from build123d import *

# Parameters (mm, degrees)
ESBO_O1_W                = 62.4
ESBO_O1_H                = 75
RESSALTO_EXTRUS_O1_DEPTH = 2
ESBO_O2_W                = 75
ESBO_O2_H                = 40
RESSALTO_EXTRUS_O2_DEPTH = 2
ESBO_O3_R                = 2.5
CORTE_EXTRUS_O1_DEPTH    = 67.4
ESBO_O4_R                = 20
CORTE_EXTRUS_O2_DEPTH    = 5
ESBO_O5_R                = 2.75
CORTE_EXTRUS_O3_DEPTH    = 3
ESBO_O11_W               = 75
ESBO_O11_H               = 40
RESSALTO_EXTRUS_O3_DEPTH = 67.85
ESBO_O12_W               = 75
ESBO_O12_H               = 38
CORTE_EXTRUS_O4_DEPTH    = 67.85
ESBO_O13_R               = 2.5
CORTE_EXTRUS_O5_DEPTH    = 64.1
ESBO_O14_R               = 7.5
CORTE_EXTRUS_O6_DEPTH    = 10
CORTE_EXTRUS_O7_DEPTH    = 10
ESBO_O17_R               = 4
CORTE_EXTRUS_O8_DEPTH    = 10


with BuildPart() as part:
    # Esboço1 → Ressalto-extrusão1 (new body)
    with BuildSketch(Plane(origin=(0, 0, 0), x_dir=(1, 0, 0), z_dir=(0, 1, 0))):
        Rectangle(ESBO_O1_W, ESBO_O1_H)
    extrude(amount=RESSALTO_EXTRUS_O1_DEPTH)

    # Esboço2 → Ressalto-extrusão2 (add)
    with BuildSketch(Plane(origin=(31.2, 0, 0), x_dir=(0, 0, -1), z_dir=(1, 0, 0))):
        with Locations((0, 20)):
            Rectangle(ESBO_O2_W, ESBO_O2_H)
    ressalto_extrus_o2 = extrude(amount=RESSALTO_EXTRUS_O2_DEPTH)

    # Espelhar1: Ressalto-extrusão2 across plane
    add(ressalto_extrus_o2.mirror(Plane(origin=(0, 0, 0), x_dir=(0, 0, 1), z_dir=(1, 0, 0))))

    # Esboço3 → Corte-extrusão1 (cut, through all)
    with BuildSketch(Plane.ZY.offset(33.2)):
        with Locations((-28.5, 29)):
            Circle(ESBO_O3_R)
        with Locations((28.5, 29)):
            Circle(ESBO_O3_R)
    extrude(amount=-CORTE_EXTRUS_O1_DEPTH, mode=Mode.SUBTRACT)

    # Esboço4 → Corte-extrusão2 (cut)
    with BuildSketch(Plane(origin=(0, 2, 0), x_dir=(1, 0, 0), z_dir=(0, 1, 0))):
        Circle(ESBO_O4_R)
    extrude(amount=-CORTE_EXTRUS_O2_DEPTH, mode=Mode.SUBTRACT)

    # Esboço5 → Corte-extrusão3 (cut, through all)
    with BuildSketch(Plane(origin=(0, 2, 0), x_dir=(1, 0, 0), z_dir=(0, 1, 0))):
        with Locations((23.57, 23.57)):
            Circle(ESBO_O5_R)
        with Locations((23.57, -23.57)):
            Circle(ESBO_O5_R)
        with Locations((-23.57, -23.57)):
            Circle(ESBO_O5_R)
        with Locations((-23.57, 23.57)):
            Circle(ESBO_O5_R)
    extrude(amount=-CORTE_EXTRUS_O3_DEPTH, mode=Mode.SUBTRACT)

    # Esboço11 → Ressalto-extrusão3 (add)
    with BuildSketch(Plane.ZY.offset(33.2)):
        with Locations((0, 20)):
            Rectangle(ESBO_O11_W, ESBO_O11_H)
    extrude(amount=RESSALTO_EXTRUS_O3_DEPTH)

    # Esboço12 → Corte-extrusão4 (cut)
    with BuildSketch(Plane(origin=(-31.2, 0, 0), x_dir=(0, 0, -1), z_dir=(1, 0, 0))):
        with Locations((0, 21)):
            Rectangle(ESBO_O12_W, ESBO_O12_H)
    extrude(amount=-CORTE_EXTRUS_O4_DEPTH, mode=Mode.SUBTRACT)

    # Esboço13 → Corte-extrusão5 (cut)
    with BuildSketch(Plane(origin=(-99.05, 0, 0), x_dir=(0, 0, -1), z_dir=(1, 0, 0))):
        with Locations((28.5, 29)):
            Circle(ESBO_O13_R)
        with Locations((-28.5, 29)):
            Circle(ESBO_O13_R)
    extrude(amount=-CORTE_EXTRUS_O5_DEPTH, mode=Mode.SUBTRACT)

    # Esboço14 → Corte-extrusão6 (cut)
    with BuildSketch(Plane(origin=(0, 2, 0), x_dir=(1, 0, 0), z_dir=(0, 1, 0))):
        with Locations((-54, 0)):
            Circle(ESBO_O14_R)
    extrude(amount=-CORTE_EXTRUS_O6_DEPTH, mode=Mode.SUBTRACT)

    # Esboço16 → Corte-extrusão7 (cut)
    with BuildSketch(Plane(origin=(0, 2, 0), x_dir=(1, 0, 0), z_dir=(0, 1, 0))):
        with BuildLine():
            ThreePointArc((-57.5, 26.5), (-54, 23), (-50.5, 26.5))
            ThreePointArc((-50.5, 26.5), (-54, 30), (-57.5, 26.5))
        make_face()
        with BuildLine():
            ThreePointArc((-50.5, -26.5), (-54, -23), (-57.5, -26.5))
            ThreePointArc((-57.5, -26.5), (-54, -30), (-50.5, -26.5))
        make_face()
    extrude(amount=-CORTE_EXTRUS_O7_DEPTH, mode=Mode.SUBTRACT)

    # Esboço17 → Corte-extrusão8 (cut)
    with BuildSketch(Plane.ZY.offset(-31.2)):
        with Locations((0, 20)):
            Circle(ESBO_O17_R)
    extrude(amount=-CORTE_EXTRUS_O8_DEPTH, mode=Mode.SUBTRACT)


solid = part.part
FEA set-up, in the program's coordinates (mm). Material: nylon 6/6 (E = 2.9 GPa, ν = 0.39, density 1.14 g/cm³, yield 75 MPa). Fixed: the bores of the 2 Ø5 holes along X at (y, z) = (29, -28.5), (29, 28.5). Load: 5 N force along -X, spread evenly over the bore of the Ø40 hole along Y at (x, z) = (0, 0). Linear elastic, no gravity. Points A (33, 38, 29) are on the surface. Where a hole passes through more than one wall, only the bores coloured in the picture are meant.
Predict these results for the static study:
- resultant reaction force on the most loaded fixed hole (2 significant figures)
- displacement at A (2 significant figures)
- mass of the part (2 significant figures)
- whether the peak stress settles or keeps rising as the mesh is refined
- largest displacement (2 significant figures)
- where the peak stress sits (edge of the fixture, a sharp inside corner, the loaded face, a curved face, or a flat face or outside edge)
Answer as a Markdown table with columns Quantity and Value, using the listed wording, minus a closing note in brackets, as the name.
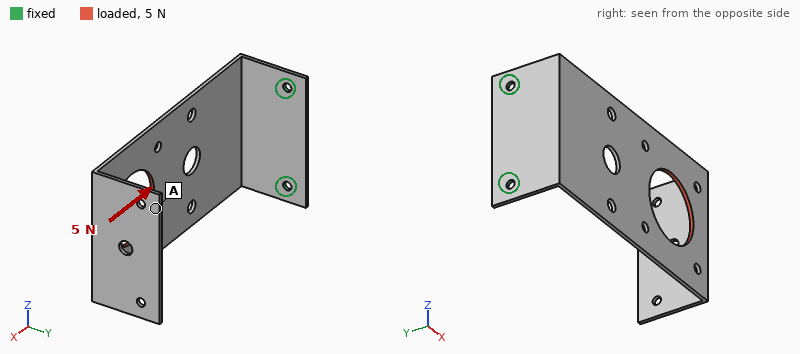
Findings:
| Quantity | Value |
|---|---|
| resultant reaction force on the most loaded fixed hole | 2.5 N |
| displacement at A | 1.9 mm |
| mass of the part | 32 g |
| whether the peak stress settles or keeps rising as the mesh is refined | keeps rising |
| largest displacement | 1.9 mm |
| where the peak stress sits | edge of the fixture |
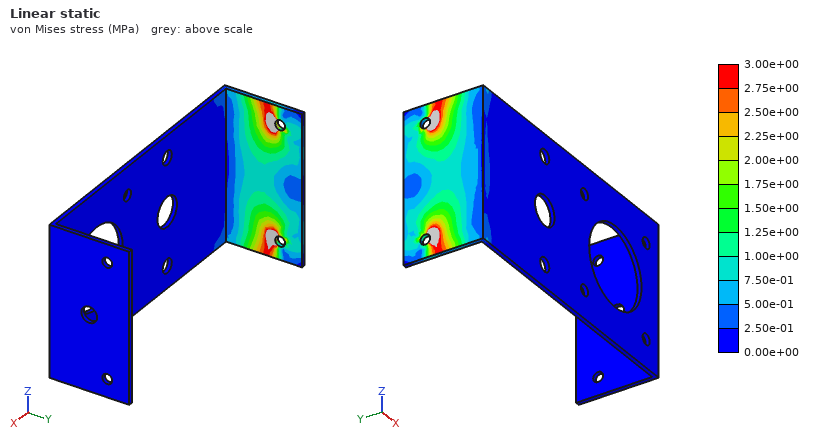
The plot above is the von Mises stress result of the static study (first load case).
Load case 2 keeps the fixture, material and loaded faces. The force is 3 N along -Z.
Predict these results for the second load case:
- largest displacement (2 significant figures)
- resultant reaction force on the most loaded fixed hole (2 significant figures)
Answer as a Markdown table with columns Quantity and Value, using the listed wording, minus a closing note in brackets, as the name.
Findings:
| Quantity | Value |
|---|---|
| largest displacement | 1.8 mm |
| resultant reaction force on the most loaded fixed hole | 5.6 N |
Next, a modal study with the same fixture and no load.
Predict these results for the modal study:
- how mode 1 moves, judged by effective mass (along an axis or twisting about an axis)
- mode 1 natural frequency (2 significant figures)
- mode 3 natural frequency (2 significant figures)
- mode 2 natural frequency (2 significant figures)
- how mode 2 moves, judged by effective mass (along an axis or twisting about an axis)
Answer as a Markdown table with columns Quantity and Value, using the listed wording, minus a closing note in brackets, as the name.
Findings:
| Quantity | Value |
|---|---|
| how mode 1 moves, judged by effective mass | along Y |
| mode 1 natural frequency | 16 Hz |
| mode 3 natural frequency | 80 Hz |
| mode 2 natural frequency | 47 Hz |
| how mode 2 moves, judged by effective mass | along Z |
